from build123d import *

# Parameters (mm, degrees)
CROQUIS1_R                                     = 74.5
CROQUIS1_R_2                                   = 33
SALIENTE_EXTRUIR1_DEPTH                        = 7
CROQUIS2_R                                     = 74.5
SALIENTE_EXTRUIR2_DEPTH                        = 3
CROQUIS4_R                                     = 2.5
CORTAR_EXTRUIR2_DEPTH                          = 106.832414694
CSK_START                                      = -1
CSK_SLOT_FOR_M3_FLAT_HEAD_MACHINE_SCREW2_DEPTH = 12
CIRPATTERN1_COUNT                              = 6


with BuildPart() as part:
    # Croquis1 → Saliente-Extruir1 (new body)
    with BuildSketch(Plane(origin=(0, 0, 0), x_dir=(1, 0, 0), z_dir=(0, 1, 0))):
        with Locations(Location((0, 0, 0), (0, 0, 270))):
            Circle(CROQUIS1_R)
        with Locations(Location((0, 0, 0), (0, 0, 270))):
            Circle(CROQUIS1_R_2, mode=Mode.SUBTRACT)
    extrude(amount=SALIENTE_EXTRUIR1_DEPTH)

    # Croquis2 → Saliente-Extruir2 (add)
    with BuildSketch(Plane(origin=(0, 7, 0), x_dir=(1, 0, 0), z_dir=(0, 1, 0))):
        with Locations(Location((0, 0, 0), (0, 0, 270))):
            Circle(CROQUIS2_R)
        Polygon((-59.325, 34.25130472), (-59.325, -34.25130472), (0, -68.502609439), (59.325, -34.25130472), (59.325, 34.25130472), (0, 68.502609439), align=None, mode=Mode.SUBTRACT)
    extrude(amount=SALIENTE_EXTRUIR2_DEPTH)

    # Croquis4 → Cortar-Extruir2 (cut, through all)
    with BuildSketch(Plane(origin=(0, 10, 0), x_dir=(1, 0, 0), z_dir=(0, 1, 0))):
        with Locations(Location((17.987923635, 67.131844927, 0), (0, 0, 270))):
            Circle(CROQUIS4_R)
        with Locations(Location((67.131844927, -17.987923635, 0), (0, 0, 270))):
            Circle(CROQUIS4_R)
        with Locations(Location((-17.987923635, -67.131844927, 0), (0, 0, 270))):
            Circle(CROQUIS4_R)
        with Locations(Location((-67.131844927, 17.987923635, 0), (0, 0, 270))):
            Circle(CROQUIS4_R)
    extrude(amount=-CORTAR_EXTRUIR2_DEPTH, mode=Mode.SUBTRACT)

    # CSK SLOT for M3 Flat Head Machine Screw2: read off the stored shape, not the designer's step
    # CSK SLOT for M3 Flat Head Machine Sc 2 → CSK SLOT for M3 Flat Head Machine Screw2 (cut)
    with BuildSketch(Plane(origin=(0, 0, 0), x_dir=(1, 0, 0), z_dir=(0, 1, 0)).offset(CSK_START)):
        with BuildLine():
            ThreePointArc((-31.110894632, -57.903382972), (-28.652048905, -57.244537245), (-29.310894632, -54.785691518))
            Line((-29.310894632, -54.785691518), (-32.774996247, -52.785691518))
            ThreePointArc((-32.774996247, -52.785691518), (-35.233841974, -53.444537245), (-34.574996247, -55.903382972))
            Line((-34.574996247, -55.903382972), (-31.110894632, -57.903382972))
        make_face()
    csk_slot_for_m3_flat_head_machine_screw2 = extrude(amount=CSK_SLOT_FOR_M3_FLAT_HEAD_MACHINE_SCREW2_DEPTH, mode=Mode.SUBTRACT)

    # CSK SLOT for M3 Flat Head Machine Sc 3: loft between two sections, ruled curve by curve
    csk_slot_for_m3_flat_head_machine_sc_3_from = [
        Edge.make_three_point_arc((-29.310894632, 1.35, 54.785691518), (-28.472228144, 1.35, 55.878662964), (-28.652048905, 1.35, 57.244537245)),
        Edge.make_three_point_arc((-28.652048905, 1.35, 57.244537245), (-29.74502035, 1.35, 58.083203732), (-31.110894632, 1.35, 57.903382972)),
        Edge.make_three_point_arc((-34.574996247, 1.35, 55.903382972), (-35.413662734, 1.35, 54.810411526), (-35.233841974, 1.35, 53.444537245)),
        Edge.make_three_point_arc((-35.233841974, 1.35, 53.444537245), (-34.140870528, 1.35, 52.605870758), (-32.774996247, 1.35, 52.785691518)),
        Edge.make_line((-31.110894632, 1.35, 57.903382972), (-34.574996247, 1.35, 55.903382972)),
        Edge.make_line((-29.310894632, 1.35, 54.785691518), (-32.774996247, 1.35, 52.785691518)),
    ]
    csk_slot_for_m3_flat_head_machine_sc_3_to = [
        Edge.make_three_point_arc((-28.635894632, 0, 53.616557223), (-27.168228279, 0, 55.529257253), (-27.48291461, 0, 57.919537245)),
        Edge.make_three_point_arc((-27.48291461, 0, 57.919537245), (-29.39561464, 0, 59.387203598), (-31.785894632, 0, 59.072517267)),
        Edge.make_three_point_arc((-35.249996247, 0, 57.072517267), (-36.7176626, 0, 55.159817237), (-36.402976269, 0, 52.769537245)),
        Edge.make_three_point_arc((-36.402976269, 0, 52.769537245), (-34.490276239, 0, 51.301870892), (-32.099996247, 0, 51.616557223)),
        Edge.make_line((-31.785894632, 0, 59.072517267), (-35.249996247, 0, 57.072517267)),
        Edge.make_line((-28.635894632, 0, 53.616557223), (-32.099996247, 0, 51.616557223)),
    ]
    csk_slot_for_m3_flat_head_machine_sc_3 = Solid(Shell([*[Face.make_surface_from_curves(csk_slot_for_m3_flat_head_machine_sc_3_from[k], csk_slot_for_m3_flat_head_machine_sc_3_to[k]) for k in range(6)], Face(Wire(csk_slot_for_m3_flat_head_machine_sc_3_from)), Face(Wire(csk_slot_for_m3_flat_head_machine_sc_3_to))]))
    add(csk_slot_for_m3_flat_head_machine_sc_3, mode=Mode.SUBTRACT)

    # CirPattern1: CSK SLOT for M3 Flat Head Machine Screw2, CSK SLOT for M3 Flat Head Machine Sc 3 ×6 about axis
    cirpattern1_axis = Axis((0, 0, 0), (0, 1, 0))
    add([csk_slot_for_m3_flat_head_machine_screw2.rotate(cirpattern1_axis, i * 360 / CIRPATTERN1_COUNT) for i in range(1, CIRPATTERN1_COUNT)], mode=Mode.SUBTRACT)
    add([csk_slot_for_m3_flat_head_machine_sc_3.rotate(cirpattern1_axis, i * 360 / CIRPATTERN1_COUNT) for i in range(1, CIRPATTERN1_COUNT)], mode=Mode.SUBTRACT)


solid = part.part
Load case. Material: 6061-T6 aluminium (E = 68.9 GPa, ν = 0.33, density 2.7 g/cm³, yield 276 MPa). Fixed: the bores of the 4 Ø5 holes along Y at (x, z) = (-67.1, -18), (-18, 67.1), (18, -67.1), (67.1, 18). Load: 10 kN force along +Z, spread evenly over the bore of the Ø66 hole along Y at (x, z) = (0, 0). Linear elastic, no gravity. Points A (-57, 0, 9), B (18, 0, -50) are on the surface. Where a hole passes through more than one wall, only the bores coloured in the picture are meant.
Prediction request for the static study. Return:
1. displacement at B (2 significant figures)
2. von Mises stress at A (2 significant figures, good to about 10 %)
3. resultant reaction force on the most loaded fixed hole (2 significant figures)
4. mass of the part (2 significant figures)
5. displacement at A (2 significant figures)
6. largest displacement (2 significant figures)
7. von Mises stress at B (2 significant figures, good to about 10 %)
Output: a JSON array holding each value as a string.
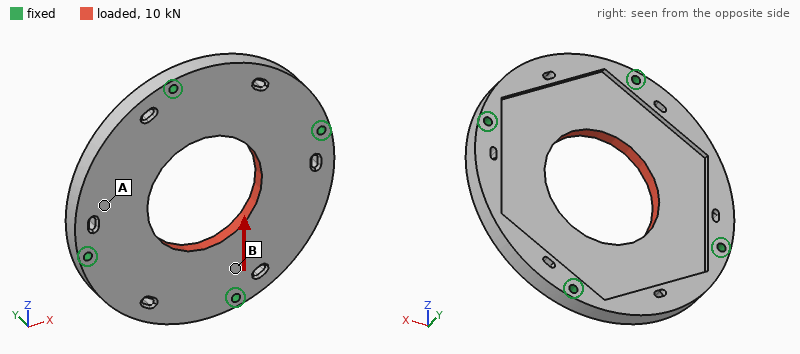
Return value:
["5.0 µm", "4.2 MPa", "2.7 kN", "300 g", "5.3 µm", "12 µm", "14 MPa"]
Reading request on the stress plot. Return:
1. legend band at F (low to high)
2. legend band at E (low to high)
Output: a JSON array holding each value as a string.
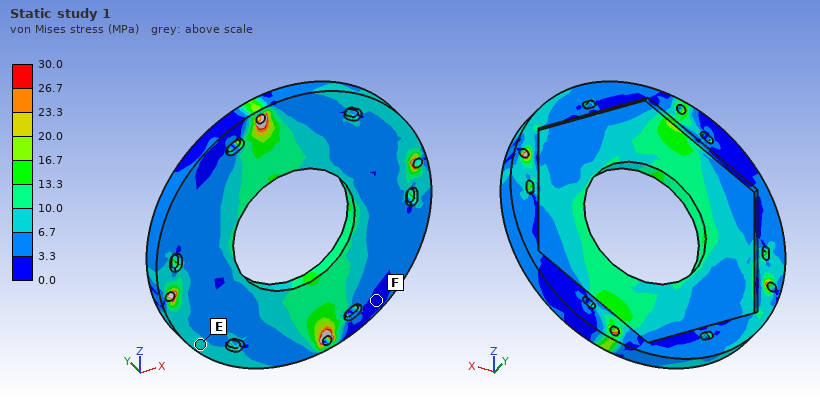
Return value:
["0.0 to 3.3 MPa", "6.7 to 10.0 MPa"]
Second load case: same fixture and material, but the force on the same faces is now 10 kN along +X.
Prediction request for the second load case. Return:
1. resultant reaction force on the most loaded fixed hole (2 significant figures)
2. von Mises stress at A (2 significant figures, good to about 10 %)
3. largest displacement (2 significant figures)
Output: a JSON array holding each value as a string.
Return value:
["2.7 kN", "6.4 MPa", "12 µm"]
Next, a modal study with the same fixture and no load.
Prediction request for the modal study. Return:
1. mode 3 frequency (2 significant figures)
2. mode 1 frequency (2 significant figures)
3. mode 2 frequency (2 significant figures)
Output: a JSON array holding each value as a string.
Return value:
["3800 Hz", "3600 Hz", "3800 Hz"]
